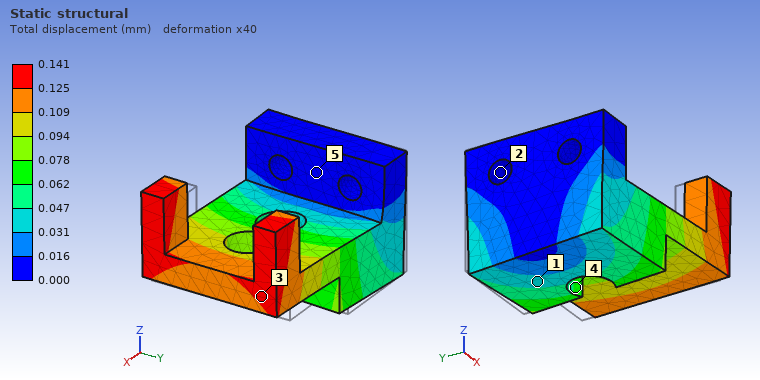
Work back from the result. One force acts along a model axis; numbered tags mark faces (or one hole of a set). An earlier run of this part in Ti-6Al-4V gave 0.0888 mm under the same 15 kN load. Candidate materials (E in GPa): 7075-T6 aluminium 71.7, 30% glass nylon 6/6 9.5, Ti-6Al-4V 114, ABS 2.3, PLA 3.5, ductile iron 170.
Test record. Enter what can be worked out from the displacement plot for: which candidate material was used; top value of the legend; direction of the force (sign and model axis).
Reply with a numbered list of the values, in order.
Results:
1. 7075-T6 aluminium
2. 0.141 mm
3. -Y
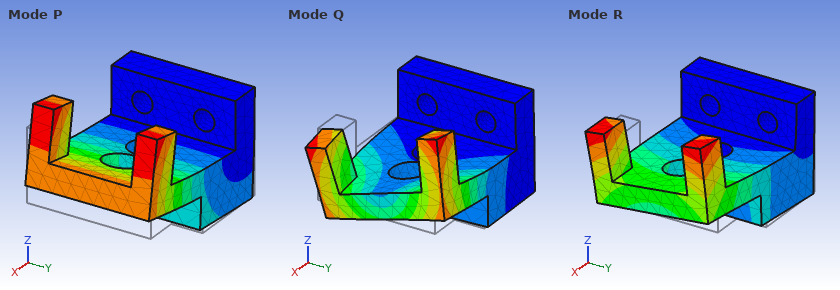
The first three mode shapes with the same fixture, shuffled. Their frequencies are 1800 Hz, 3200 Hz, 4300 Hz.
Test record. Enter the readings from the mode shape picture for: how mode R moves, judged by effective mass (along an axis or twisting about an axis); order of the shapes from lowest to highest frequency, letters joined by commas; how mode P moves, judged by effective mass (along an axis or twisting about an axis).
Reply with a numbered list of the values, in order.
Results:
1. along Y
2. P, R, Q
3. along Z
